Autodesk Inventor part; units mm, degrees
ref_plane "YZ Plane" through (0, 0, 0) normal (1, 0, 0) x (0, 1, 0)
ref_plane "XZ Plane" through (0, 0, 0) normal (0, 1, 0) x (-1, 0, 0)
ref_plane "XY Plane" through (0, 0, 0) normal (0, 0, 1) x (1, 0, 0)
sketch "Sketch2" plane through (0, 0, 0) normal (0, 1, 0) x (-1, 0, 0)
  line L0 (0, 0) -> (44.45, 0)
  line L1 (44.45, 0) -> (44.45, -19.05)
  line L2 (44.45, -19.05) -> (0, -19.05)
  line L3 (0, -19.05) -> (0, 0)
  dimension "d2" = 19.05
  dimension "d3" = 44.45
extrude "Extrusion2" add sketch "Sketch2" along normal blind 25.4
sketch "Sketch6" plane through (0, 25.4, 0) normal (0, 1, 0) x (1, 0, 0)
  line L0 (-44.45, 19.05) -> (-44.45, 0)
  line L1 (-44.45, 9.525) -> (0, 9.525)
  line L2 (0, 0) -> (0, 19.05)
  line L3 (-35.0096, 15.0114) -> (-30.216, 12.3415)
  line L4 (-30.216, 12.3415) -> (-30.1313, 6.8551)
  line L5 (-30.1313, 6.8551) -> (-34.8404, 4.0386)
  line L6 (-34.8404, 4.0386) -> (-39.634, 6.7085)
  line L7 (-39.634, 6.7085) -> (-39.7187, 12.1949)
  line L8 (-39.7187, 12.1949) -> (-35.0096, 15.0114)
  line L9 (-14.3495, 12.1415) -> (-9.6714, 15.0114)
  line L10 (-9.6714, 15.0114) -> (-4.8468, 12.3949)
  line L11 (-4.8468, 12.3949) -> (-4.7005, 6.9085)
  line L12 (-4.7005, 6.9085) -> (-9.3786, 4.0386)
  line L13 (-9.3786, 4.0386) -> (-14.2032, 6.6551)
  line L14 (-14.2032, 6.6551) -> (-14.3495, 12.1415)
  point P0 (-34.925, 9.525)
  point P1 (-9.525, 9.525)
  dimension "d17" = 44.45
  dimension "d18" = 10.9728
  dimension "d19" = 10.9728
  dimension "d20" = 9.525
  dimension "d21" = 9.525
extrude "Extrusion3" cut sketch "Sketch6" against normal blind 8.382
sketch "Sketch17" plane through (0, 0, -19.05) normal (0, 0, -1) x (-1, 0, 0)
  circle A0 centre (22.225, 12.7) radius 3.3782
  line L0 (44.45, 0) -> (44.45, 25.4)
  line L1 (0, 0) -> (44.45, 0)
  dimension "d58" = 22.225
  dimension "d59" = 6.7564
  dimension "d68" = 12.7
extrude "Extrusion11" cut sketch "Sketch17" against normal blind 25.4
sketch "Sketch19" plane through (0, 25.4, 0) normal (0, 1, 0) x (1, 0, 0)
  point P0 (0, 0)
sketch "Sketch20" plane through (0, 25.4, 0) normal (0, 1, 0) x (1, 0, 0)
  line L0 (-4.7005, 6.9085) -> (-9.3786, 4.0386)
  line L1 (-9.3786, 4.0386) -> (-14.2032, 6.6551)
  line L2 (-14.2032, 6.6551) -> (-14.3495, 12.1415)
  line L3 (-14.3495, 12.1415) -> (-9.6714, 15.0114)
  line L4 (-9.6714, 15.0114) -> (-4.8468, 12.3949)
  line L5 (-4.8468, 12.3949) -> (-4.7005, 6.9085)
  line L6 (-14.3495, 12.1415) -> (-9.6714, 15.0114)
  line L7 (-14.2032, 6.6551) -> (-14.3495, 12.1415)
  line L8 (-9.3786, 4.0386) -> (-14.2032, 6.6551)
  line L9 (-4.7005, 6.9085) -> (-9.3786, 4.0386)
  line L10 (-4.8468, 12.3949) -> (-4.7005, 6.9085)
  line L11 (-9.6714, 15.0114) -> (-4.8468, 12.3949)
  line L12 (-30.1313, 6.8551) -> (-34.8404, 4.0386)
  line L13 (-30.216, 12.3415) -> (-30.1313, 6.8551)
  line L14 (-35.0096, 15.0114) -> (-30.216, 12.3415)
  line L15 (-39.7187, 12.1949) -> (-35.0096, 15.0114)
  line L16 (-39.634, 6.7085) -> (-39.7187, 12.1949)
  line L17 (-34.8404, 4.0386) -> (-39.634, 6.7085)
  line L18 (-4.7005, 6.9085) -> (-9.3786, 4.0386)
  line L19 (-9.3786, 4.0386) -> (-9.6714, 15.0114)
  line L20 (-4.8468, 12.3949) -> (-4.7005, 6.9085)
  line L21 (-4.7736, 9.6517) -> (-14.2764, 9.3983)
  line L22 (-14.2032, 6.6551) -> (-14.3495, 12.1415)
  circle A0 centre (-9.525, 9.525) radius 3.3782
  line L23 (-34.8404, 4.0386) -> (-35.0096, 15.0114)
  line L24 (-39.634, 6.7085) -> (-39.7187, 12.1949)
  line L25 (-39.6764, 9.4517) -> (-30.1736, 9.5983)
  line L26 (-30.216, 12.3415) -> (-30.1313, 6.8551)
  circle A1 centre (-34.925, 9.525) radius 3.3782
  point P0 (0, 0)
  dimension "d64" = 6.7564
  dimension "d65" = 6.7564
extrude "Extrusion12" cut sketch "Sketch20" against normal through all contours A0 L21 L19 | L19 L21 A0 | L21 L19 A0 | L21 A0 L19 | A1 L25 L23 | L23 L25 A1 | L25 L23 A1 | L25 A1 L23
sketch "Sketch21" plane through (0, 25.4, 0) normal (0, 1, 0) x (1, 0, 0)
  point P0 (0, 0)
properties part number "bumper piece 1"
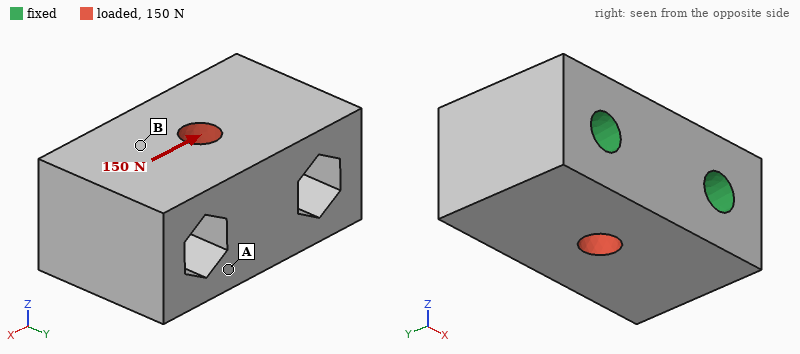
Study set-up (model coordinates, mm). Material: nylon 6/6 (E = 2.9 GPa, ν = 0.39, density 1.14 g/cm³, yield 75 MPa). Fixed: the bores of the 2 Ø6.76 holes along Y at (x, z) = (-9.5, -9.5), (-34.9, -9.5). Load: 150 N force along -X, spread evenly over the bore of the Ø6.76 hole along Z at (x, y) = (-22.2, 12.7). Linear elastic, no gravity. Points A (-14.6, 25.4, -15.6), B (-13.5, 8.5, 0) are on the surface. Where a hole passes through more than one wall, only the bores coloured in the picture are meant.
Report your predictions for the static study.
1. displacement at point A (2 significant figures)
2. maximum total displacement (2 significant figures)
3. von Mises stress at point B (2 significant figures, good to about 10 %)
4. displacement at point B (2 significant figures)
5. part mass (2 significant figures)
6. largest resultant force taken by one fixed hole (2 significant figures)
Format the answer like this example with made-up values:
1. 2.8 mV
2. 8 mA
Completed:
1. 0.84 µm
2. 1.6 µm
3. 0.18 MPa
4. 0.63 µm
5. 21 g
6. 76 N
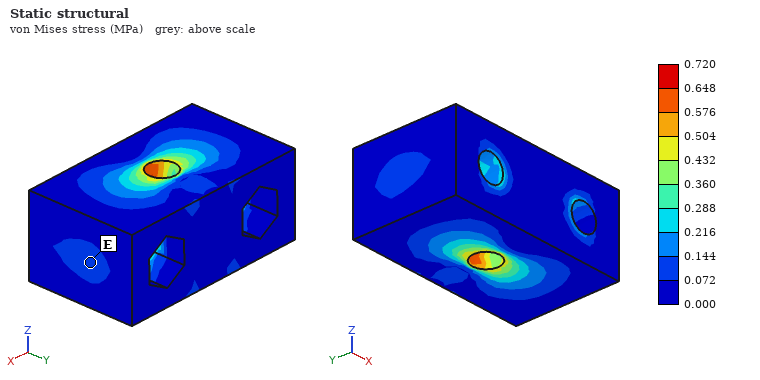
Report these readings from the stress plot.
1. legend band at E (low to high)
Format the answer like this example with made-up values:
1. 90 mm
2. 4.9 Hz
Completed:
1. 0.072 to 0.144 MPa
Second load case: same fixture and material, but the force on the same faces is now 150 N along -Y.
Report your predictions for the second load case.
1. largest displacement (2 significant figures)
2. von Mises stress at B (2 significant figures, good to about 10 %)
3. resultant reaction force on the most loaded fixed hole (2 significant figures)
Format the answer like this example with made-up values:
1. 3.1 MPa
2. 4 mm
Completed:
1. 2.7 µm
2. 0.25 MPa
3. 77 N
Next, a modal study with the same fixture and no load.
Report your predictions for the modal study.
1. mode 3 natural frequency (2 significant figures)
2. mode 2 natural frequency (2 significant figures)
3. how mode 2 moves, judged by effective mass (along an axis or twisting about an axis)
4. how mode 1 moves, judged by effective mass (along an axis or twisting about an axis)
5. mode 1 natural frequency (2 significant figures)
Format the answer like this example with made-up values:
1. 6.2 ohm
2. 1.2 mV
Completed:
1. 13 kHz
2. 12 kHz
3. twisting about Y
4. along Z
5. 9700 Hz
